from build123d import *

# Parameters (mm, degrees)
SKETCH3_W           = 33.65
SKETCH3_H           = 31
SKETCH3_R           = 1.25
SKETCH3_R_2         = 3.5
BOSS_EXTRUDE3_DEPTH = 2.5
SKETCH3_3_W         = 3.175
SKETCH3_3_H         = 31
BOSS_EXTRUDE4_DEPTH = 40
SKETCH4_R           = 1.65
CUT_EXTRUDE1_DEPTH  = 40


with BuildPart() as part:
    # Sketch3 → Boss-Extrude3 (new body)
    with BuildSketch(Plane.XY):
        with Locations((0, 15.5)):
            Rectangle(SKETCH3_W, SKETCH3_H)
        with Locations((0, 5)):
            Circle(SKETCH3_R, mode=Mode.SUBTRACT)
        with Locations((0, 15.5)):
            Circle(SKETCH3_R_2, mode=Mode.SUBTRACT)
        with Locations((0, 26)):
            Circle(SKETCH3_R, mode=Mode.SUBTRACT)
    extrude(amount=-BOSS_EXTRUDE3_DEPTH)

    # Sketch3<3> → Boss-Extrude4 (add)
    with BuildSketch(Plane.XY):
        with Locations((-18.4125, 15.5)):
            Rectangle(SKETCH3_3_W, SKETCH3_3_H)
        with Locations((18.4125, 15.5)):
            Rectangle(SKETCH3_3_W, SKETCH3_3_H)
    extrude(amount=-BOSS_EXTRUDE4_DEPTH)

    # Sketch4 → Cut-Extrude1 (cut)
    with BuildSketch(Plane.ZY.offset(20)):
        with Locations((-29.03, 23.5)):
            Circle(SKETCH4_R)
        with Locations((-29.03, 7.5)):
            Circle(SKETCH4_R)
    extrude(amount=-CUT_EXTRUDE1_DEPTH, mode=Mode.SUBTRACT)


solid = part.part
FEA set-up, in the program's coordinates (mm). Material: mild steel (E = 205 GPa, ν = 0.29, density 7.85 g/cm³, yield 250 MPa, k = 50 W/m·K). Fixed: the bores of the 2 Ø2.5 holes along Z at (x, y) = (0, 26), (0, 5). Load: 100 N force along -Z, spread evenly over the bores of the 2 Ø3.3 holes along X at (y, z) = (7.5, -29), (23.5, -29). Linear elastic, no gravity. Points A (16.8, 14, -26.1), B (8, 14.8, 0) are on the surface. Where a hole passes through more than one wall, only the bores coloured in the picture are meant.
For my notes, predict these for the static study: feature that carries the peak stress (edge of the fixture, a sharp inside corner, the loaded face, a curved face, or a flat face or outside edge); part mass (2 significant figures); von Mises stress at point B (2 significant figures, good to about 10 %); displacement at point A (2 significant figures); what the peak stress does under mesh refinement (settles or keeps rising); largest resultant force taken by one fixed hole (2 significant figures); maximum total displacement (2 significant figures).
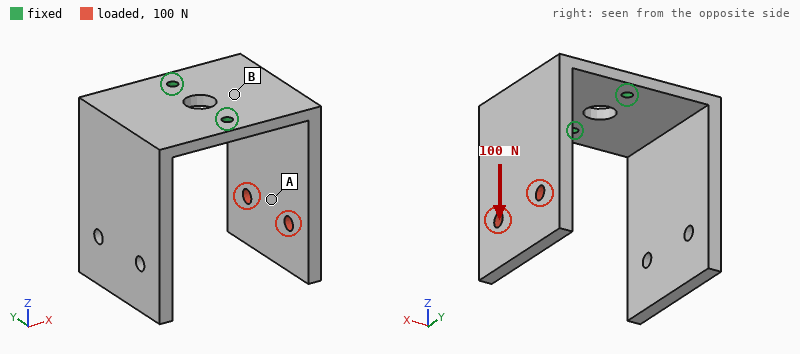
edge of the fixture
80 g
24 MPa
61 µm
keeps rising
50 N
93 µm
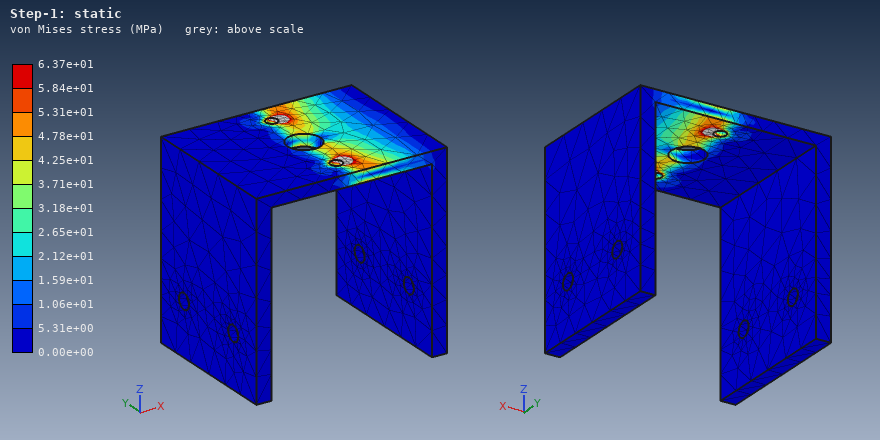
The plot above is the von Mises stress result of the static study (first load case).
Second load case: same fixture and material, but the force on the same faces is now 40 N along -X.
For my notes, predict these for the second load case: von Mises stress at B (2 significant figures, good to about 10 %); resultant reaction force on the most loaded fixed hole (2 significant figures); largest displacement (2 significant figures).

25 MPa
21 N
0.12 mm
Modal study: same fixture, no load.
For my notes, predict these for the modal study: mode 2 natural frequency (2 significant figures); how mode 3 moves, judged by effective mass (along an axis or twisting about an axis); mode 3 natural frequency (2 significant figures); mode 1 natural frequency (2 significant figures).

760 Hz
twisting about Z
1500 Hz
730 Hz
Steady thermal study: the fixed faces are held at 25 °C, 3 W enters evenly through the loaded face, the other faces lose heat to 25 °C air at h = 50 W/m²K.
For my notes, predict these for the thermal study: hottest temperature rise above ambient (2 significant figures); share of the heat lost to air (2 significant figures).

17 K
64 %
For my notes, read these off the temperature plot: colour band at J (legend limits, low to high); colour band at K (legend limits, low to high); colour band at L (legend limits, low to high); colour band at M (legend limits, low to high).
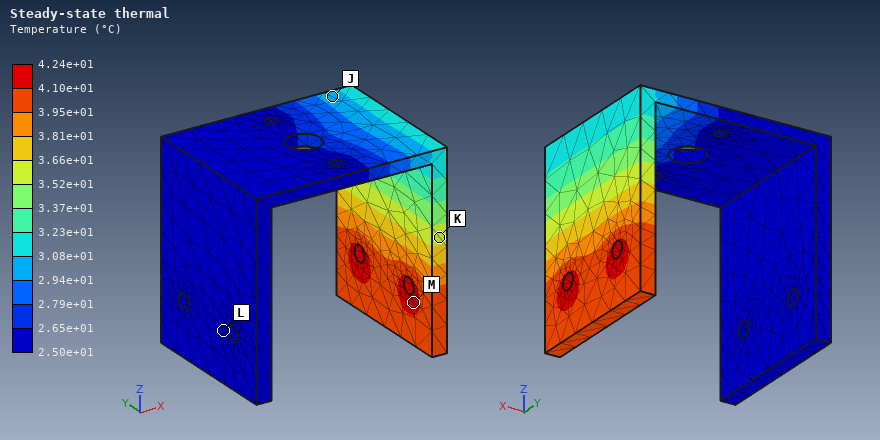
2.94e+01 to 3.08e+01 °C
3.52e+01 to 3.66e+01 °C
2.50e+01 to 2.65e+01 °C
4.10e+01 to 4.24e+01 °C
